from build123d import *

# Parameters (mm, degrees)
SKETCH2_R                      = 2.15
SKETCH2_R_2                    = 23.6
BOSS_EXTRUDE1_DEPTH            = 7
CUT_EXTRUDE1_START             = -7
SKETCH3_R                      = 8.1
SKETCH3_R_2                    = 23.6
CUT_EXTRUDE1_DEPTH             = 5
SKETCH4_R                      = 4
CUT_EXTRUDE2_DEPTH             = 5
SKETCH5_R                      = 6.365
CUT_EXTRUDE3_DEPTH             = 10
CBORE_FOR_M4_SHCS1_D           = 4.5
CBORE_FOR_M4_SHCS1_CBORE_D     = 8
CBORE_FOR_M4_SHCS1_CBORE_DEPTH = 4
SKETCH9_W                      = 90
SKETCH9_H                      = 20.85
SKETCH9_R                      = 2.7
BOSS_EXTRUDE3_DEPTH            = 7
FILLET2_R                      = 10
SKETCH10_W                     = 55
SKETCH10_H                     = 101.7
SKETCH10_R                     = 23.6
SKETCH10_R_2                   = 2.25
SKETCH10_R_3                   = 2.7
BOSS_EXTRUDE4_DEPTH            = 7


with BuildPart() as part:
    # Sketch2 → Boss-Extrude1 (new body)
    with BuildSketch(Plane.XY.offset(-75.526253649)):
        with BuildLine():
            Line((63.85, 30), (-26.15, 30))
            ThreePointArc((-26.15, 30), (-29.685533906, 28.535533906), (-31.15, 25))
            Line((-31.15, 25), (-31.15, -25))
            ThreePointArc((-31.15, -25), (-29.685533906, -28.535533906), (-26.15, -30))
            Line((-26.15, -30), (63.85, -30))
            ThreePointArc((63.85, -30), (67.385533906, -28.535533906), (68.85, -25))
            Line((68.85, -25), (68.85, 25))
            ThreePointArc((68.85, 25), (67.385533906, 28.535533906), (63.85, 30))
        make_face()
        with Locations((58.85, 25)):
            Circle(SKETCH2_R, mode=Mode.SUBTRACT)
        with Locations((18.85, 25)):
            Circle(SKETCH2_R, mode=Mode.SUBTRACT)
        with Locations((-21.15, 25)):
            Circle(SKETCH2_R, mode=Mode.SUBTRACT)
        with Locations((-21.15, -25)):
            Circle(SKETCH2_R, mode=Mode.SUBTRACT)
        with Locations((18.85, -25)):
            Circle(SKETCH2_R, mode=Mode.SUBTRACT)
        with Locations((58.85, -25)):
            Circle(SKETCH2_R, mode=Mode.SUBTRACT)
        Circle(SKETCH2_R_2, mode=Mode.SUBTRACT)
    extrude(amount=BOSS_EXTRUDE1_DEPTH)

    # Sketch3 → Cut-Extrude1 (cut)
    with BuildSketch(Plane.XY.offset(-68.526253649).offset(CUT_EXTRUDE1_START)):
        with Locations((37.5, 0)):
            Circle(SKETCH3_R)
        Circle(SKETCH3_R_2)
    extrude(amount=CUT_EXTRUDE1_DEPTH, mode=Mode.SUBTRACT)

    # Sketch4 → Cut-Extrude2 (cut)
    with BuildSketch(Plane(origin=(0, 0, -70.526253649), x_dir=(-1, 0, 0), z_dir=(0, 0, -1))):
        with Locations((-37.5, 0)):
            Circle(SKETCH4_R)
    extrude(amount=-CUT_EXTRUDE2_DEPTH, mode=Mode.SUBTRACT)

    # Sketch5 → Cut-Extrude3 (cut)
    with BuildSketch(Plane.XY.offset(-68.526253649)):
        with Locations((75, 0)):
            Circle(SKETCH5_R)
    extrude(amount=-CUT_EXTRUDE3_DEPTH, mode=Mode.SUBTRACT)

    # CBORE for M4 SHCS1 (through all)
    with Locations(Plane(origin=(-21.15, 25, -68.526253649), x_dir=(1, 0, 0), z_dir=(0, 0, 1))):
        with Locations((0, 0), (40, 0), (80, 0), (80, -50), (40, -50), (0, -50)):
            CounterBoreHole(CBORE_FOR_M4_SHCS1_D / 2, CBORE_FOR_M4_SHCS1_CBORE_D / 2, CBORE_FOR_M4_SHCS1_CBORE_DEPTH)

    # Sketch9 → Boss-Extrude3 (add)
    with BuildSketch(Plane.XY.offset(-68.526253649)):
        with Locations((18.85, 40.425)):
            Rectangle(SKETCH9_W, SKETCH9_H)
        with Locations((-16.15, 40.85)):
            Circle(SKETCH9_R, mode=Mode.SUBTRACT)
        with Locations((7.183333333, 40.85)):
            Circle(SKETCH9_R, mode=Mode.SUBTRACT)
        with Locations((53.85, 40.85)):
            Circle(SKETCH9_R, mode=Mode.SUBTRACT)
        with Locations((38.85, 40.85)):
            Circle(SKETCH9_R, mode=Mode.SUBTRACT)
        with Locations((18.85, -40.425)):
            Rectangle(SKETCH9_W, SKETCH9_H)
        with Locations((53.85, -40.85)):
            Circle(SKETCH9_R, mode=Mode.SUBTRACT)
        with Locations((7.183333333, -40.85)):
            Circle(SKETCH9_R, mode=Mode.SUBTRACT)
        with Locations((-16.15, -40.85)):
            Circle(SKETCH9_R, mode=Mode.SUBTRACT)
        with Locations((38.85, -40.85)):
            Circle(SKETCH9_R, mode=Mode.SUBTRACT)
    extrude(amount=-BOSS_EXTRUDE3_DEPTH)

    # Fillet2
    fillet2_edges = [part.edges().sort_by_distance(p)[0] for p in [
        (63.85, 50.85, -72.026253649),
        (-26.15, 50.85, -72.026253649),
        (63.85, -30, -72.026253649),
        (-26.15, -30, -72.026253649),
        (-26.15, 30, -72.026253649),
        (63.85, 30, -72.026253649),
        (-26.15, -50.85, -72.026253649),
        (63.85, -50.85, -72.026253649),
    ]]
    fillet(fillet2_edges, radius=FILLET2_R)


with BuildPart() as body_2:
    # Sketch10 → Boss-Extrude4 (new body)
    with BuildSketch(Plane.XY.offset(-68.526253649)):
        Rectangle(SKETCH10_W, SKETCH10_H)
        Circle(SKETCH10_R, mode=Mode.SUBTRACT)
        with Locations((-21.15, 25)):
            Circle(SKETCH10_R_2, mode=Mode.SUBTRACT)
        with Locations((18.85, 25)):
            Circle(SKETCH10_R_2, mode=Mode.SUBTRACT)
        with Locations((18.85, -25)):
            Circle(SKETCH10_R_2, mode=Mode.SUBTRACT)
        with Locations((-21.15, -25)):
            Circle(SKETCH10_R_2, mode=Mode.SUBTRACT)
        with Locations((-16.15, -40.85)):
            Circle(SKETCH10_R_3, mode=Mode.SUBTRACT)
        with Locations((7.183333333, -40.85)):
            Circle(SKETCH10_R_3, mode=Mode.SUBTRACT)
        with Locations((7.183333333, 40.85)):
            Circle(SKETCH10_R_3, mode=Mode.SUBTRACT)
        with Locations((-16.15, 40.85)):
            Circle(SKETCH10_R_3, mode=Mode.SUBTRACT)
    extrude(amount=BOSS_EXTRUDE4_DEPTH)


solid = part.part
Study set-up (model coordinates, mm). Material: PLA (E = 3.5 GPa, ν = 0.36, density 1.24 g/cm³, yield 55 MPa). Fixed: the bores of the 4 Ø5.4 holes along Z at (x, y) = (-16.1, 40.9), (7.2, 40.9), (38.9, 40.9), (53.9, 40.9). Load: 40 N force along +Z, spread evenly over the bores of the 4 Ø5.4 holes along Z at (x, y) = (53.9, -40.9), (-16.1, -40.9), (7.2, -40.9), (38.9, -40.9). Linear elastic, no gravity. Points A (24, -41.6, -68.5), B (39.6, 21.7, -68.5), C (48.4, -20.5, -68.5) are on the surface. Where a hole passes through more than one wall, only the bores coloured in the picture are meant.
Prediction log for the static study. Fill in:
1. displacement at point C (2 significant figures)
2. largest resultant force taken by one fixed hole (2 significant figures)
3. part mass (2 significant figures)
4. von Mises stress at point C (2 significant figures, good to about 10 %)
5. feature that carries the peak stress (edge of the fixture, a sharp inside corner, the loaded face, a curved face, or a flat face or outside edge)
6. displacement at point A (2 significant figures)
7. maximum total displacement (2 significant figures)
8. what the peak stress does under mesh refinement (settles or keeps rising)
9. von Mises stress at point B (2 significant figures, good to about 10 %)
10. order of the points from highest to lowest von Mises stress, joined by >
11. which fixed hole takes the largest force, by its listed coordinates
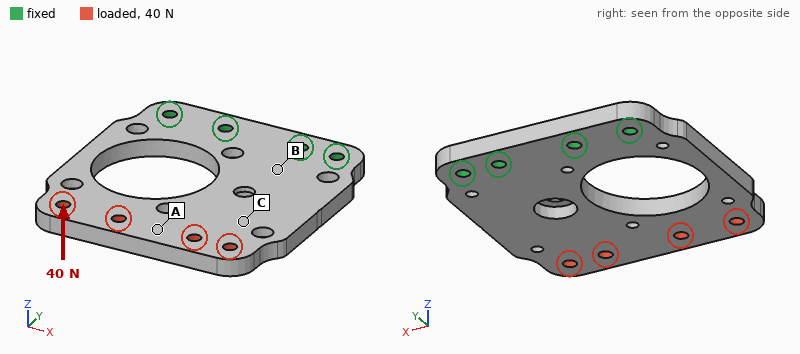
0.74 mm
33 N
64 g
2.0 MPa
edge of the fixture
1.3 mm
1.5 mm
keeps rising
4.6 MPa
B > C > A
(38.9, 40.9)
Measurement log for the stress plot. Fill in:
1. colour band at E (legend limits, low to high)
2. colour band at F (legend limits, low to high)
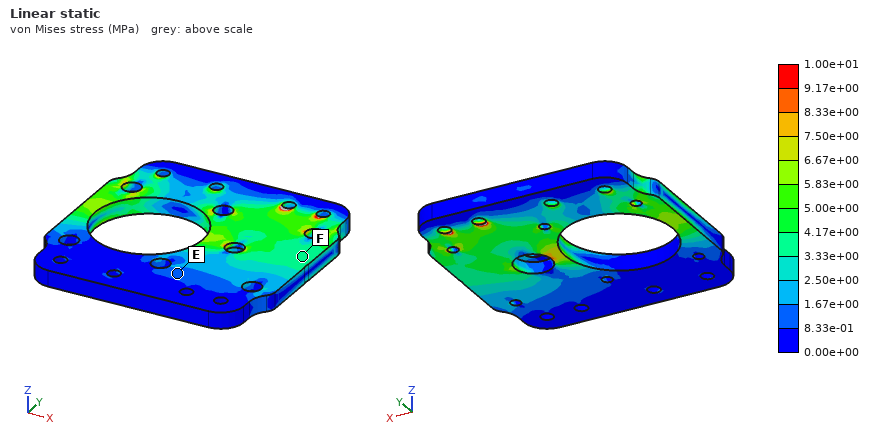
8.33e-01 to 1.67e+00 MPa
3.33e+00 to 4.17e+00 MPa
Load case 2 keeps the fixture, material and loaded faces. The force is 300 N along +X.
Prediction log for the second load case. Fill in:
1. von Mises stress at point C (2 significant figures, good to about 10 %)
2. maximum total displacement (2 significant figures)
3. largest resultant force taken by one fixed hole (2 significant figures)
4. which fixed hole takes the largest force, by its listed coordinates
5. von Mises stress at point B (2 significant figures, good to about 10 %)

0.94 MPa
0.22 mm
420 N
(53.9, 40.9)
1.7 MPa
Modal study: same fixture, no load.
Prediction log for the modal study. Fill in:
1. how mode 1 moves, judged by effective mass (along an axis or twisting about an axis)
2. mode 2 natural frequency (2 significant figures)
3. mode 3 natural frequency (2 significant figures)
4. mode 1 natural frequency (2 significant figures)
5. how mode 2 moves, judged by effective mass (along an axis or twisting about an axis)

along Z
470 Hz
1200 Hz
200 Hz
twisting about Y
